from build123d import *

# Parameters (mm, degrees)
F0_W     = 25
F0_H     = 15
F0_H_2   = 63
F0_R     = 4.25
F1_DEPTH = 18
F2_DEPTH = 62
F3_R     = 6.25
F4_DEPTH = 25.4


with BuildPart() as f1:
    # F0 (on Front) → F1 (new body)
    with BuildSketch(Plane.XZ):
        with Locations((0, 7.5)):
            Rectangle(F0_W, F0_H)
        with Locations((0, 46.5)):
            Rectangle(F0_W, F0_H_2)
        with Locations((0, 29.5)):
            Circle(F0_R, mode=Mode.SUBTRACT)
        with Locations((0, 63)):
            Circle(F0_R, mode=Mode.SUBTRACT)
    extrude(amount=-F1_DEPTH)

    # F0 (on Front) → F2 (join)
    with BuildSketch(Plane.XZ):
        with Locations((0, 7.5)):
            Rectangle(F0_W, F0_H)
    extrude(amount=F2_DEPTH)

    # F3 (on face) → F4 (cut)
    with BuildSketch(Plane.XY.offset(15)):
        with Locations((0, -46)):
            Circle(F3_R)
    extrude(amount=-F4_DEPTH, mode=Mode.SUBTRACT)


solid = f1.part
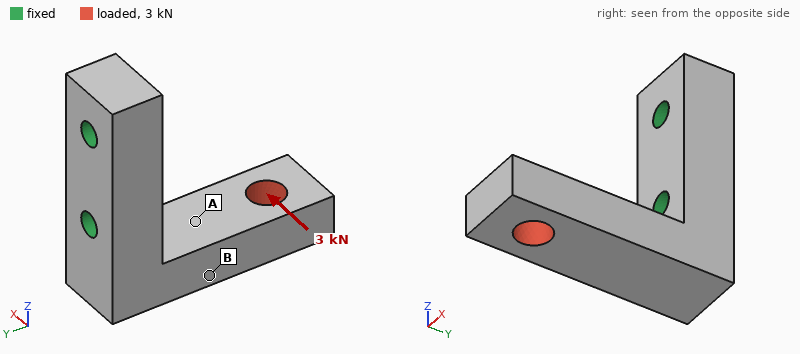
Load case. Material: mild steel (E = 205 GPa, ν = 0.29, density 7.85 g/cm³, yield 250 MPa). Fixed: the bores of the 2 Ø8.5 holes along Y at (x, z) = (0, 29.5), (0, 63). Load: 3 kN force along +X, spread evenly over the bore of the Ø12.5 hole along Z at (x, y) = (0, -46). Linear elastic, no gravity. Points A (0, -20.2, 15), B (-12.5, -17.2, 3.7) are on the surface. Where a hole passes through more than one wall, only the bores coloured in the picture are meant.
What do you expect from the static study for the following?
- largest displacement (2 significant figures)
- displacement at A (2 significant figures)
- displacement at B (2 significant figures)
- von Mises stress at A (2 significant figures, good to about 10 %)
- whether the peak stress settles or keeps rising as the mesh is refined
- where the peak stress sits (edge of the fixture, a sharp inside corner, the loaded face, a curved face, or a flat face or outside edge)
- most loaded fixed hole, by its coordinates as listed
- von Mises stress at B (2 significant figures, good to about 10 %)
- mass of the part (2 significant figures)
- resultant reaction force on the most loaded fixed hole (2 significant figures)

0.16 mm
0.053 mm
0.054 mm
23 MPa
keeps rising
edge of the fixture
(0, 29.5)
55 MPa
430 g
3.8 kN
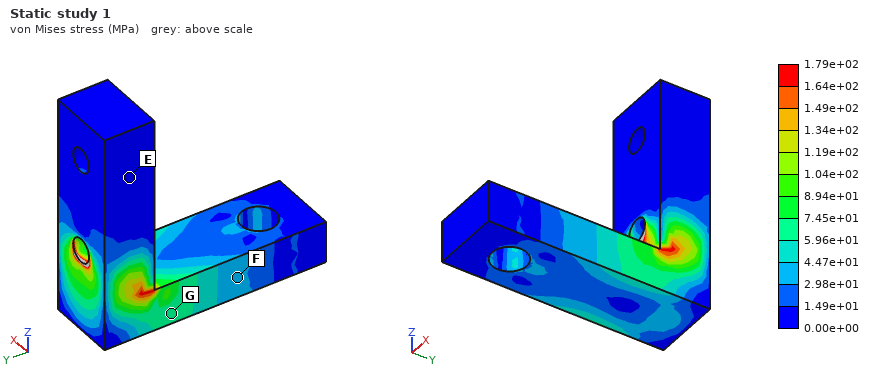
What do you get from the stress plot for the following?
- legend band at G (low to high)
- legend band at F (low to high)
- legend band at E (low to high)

5.96e+01 to 7.45e+01 MPa
2.98e+01 to 4.47e+01 MPa
0.00e+00 to 1.49e+01 MPa
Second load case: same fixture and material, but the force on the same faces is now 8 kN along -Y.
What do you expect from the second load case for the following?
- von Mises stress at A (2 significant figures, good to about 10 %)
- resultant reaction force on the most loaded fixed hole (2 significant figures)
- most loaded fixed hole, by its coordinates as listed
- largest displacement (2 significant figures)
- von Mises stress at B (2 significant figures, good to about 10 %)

20 MPa
8.6 kN
(0, 29.5)
66 µm
21 MPa
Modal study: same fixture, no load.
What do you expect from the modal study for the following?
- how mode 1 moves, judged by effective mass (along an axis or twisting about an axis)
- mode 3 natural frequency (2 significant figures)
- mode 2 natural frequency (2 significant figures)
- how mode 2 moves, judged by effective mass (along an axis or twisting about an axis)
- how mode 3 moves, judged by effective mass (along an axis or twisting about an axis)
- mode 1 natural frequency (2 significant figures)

along Z
8100 Hz
2500 Hz
along X
along Y
2100 Hz
